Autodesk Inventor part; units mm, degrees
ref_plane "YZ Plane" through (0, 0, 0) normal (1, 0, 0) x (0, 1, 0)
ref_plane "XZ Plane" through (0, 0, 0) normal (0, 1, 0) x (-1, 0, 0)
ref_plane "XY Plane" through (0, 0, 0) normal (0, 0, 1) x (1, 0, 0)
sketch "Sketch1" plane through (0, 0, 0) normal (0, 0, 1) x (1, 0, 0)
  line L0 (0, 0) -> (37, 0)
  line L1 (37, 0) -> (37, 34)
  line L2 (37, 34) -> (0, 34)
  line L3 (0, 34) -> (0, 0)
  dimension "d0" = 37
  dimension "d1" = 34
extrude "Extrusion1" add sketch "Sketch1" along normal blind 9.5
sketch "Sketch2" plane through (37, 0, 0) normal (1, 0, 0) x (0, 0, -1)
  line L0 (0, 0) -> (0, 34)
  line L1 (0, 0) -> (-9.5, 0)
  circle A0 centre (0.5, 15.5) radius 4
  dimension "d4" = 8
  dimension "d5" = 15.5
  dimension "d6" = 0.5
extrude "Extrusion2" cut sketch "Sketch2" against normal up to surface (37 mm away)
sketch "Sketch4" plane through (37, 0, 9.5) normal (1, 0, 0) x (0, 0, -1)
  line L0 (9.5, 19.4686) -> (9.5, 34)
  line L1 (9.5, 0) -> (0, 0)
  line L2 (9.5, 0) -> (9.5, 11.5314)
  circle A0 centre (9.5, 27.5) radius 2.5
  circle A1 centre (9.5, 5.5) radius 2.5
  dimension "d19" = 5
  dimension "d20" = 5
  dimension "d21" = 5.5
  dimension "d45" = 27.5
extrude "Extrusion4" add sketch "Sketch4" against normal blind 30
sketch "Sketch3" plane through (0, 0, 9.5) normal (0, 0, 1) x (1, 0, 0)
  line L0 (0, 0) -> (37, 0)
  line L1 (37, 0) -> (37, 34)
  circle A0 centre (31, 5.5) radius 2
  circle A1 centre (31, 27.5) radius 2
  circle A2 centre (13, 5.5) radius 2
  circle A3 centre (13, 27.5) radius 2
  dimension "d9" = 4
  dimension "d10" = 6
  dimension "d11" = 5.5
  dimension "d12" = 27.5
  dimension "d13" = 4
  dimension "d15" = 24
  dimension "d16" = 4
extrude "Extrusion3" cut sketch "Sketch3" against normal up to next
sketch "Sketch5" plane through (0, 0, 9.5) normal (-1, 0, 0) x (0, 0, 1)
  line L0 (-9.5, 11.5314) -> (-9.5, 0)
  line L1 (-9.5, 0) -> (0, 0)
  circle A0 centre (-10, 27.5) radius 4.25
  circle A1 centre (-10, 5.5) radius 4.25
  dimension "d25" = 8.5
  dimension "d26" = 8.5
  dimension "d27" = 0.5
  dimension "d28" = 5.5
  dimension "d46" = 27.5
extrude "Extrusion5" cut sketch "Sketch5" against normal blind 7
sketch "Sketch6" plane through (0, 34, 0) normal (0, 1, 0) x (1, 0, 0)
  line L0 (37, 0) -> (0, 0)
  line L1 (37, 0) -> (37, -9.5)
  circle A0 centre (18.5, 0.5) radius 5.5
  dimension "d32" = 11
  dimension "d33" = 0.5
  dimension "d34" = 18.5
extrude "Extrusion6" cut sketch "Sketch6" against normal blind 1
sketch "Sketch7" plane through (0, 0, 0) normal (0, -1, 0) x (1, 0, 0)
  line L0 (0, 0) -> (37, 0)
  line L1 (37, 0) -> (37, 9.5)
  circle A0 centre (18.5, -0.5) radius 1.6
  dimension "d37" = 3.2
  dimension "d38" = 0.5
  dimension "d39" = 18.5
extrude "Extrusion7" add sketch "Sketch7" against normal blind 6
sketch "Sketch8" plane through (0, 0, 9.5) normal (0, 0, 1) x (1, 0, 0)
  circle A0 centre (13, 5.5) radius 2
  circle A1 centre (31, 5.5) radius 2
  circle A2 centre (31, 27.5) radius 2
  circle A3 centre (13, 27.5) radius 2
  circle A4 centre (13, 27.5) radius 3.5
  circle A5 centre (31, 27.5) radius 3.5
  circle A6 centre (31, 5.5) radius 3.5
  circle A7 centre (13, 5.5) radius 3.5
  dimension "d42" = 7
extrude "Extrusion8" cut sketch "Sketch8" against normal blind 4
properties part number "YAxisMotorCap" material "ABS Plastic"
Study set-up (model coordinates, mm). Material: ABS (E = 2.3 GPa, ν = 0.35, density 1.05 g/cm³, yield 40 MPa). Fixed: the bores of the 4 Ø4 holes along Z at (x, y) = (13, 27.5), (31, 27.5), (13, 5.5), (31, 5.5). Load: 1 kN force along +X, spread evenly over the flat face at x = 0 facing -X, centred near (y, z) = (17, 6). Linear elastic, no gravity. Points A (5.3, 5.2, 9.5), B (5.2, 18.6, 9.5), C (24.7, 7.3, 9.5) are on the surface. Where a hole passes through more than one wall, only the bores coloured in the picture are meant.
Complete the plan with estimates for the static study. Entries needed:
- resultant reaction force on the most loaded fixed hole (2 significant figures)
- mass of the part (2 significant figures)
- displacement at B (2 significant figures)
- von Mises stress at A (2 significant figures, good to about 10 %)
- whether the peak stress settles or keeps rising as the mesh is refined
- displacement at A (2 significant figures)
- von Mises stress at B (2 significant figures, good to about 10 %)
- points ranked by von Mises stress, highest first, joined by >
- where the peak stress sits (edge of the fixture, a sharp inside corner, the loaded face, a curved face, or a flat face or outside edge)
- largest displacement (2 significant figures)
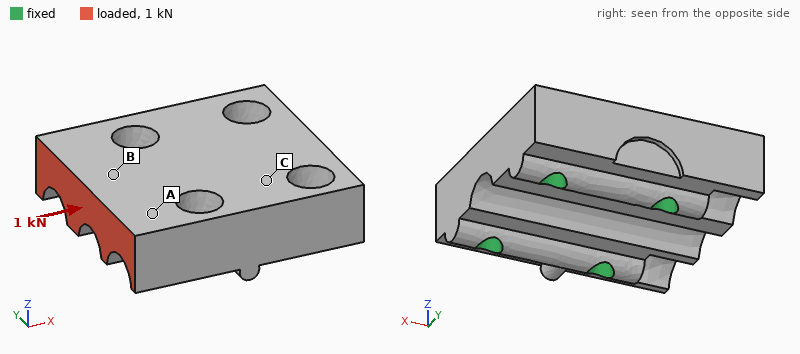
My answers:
390 N
11 g
51 µm
2.5 MPa
keeps rising
50 µm
4.3 MPa
B > A > C
edge of the fixture
70 µm
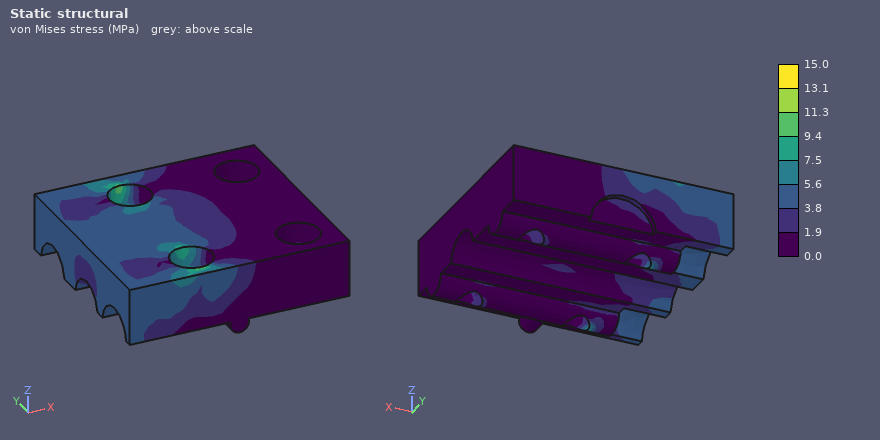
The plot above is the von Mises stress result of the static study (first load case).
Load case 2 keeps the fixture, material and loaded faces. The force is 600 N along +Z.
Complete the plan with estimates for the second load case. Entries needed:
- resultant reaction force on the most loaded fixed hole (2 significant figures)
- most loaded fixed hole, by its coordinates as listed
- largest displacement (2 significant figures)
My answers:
460 N
(13, 27.5)
0.25 mm
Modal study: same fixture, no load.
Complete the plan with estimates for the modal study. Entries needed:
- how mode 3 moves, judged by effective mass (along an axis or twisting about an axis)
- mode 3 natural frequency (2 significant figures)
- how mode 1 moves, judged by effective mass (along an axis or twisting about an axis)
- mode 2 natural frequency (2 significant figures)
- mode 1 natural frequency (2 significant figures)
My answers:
along Y
13 kHz
along Z
10 kHz
7700 Hz
